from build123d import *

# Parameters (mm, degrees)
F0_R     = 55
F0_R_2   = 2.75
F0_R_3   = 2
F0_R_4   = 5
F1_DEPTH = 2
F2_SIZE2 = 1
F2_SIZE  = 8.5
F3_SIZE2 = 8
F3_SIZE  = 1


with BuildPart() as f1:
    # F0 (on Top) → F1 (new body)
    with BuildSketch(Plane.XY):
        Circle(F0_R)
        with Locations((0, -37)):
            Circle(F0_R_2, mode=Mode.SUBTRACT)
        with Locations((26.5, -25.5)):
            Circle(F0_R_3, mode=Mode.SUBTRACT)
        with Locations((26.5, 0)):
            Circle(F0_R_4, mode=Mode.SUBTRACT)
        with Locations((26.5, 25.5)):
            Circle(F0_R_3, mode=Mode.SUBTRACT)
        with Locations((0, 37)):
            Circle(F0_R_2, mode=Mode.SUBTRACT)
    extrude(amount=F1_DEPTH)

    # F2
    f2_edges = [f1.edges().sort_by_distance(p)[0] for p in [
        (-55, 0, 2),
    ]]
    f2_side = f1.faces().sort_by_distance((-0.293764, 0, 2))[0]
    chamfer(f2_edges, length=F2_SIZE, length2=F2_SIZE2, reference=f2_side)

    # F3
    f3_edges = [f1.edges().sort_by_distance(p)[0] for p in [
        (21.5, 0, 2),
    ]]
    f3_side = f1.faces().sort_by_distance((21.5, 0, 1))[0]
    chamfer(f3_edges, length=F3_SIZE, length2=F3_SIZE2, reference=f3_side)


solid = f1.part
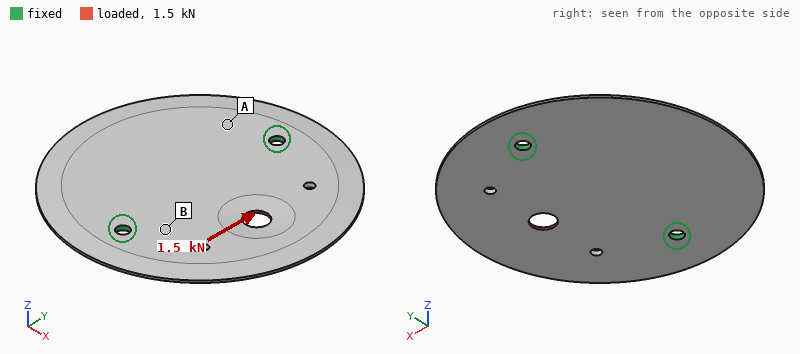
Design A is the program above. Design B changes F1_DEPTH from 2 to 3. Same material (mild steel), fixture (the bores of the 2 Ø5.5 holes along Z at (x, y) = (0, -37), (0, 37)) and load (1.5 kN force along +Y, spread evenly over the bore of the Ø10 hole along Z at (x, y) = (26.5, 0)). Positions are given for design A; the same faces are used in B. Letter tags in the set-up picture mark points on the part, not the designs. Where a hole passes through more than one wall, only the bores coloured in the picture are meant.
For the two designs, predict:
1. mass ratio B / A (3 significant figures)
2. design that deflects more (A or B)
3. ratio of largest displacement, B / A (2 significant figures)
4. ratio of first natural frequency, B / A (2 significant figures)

1.55
A
0.34
1.4
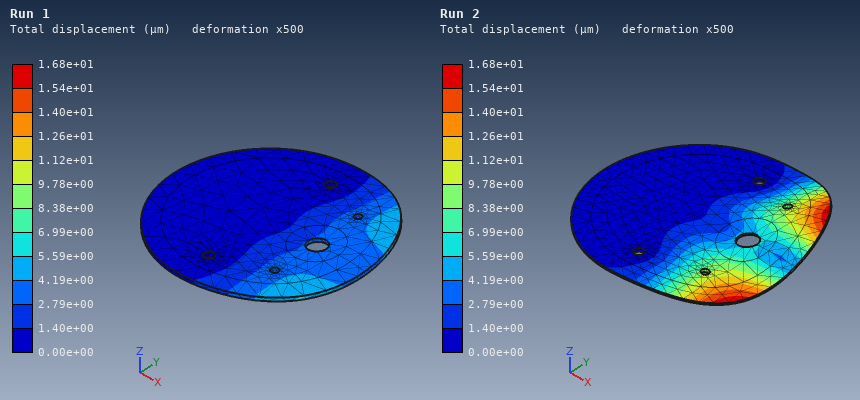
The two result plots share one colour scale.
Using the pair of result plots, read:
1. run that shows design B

Run 1
